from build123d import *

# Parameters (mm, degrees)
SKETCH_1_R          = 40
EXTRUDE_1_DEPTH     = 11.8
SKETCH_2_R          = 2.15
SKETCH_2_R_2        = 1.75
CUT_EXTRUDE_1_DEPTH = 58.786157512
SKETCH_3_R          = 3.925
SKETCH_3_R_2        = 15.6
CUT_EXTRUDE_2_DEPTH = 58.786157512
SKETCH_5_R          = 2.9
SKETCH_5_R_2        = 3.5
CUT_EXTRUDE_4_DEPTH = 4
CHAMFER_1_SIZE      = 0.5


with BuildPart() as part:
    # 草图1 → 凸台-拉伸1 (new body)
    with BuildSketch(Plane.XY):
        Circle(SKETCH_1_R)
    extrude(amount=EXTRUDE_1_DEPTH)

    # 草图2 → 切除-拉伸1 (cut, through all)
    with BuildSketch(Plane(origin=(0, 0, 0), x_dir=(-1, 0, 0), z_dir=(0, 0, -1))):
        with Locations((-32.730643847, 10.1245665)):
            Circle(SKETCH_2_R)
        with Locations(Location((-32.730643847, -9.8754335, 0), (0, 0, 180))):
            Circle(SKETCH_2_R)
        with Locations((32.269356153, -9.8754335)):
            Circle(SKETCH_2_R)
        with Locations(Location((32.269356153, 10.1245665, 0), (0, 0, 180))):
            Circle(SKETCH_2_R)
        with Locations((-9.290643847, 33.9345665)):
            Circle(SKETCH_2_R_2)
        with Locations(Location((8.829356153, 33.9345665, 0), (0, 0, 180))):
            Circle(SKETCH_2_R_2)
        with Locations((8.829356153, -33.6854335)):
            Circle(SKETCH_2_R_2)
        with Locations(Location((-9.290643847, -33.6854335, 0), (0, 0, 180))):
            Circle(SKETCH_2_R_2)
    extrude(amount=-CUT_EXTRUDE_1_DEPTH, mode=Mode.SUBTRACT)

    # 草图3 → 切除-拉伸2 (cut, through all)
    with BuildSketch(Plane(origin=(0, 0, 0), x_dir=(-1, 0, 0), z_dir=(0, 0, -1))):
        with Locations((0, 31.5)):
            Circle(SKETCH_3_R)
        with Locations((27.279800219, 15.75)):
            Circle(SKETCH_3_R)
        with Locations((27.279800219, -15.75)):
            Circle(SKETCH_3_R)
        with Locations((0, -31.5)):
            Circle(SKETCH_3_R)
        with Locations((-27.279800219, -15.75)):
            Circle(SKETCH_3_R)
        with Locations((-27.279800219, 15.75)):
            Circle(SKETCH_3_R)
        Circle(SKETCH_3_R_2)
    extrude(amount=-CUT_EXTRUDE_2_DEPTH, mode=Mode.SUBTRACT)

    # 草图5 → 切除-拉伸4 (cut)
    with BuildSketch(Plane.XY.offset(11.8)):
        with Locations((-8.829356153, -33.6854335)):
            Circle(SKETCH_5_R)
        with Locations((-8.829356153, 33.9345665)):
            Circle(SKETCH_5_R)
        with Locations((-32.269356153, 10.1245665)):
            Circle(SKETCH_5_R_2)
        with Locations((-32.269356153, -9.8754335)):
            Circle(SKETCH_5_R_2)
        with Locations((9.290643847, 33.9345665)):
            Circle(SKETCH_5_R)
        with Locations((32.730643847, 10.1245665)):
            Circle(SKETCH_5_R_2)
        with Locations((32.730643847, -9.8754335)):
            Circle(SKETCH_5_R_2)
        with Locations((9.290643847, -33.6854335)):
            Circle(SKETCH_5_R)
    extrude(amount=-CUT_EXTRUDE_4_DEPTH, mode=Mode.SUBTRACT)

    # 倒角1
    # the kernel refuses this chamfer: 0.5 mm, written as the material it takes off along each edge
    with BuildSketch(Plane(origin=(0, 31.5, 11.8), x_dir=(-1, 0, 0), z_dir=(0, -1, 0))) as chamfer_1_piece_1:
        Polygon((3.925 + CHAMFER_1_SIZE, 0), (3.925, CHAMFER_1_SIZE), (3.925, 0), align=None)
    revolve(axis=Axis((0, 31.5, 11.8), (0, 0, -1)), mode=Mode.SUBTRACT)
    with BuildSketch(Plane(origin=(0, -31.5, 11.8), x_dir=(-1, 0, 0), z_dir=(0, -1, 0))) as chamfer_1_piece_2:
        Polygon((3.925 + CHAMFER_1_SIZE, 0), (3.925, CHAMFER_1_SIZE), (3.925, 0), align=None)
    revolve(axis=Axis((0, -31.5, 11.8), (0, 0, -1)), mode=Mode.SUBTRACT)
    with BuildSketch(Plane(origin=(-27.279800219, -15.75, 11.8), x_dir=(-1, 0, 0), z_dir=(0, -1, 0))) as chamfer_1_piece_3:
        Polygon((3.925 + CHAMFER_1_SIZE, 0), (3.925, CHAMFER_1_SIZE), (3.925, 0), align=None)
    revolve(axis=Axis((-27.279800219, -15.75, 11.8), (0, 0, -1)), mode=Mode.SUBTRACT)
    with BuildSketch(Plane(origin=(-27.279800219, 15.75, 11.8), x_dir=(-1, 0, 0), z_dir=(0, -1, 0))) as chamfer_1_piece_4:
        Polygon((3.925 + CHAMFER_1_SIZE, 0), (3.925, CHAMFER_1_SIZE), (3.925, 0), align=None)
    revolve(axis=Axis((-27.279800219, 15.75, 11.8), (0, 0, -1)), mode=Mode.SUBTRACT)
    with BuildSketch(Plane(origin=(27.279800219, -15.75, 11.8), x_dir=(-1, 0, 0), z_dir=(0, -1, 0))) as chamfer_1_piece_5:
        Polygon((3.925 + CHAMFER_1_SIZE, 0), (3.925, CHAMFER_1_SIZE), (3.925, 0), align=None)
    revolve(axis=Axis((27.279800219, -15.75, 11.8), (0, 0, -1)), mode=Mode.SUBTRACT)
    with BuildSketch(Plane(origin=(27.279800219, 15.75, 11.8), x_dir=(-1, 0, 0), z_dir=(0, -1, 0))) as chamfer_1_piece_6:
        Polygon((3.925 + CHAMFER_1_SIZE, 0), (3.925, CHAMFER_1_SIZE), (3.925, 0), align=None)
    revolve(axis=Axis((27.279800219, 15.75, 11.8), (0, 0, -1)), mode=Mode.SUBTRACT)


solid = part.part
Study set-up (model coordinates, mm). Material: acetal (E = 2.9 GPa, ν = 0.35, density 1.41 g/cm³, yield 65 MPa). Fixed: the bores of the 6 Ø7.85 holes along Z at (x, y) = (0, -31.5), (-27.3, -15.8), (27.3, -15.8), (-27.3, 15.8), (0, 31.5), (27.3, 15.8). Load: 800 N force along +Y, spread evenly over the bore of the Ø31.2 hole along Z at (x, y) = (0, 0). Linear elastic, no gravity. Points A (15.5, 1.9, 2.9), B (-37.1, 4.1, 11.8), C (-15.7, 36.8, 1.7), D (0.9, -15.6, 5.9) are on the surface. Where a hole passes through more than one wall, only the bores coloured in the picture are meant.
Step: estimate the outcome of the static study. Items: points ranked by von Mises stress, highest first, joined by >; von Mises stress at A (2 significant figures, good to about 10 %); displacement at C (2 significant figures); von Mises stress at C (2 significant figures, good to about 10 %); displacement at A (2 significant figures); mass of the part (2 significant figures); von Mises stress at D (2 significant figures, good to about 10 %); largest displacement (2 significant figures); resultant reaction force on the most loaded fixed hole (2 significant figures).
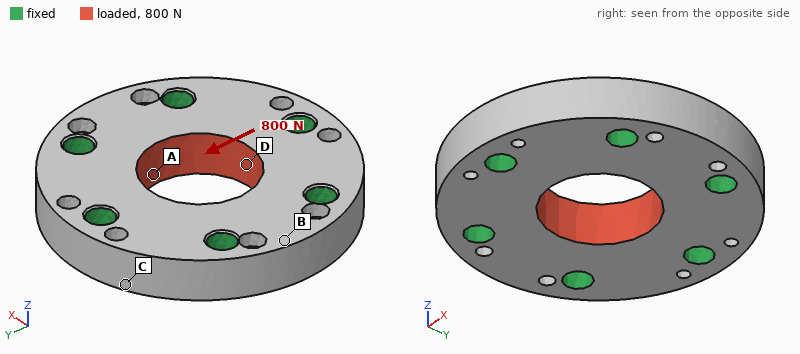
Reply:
A > D > C > B
1.2 MPa
2.1 µm
0.36 MPa
4.7 µm
64 g
0.74 MPa
5.2 µm
190 N
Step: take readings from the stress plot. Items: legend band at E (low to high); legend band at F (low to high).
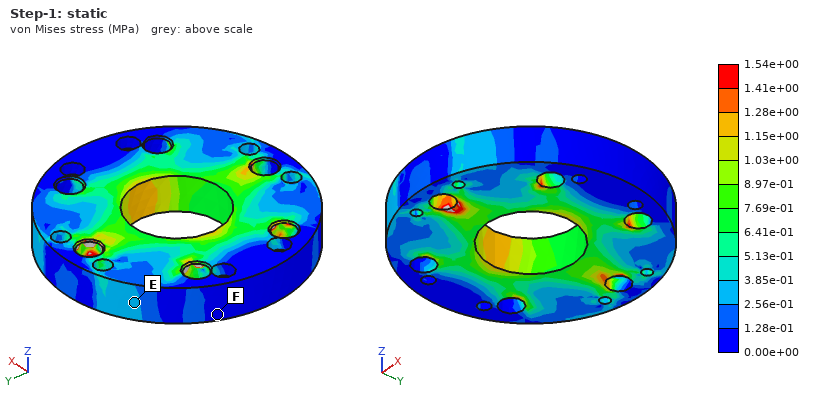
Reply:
2.56e-01 to 3.85e-01 MPa
0.00e+00 to 1.28e-01 MPa
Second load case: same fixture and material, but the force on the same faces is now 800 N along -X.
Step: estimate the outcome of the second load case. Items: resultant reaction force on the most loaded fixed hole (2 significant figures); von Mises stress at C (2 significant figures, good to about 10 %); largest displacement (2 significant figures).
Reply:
170 N
0.17 MPa
5.8 µm
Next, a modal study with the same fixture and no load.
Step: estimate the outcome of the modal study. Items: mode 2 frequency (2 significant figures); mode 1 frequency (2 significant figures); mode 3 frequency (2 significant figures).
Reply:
9000 Hz
8800 Hz
9200 Hz
